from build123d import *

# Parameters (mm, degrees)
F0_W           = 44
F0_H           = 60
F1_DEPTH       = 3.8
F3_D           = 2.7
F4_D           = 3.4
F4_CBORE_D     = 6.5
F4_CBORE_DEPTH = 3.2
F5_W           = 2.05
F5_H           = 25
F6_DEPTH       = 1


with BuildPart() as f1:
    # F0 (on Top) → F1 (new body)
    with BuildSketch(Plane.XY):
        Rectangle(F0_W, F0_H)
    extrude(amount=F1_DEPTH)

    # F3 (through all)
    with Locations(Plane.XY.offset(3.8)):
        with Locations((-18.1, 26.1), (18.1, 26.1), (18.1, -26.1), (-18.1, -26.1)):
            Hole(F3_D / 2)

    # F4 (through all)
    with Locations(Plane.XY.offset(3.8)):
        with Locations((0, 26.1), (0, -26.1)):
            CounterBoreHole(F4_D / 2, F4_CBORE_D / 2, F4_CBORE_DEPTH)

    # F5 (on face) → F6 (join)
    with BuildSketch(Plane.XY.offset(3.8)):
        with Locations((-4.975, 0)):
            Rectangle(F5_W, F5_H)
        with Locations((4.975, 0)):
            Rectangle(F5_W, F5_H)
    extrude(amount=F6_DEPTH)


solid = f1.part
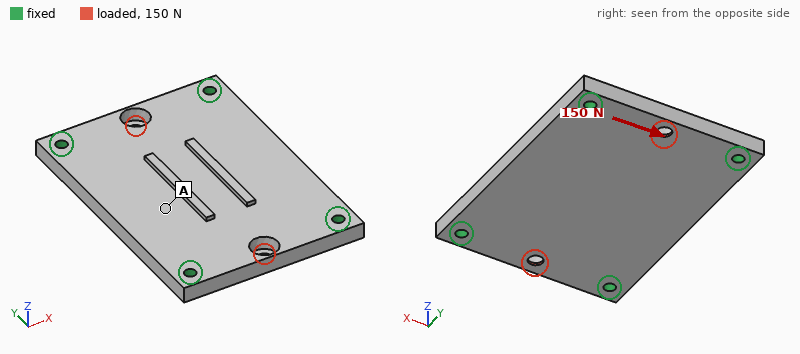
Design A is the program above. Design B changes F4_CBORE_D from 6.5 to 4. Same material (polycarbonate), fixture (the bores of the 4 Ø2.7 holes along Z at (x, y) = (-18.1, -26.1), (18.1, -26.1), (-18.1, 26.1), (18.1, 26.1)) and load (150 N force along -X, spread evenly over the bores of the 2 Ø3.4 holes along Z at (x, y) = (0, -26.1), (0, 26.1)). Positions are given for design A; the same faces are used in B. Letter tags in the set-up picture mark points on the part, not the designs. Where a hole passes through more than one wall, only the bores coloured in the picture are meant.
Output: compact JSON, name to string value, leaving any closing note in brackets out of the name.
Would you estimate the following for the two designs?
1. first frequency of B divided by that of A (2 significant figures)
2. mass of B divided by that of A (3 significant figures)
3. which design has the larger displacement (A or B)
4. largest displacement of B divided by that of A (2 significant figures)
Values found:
{"first frequency of B divided by that of A": "1.0", "mass of B divided by that of A": "1.01", "which design has the larger displacement": "A", "largest displacement of B divided by that of A": "0.78"}
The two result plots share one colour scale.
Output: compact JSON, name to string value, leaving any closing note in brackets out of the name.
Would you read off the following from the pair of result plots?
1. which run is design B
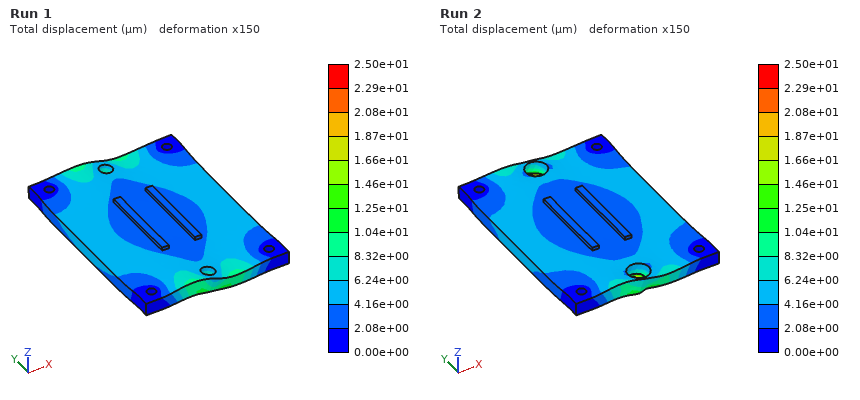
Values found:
{"which run is design B": "Run 1"}
